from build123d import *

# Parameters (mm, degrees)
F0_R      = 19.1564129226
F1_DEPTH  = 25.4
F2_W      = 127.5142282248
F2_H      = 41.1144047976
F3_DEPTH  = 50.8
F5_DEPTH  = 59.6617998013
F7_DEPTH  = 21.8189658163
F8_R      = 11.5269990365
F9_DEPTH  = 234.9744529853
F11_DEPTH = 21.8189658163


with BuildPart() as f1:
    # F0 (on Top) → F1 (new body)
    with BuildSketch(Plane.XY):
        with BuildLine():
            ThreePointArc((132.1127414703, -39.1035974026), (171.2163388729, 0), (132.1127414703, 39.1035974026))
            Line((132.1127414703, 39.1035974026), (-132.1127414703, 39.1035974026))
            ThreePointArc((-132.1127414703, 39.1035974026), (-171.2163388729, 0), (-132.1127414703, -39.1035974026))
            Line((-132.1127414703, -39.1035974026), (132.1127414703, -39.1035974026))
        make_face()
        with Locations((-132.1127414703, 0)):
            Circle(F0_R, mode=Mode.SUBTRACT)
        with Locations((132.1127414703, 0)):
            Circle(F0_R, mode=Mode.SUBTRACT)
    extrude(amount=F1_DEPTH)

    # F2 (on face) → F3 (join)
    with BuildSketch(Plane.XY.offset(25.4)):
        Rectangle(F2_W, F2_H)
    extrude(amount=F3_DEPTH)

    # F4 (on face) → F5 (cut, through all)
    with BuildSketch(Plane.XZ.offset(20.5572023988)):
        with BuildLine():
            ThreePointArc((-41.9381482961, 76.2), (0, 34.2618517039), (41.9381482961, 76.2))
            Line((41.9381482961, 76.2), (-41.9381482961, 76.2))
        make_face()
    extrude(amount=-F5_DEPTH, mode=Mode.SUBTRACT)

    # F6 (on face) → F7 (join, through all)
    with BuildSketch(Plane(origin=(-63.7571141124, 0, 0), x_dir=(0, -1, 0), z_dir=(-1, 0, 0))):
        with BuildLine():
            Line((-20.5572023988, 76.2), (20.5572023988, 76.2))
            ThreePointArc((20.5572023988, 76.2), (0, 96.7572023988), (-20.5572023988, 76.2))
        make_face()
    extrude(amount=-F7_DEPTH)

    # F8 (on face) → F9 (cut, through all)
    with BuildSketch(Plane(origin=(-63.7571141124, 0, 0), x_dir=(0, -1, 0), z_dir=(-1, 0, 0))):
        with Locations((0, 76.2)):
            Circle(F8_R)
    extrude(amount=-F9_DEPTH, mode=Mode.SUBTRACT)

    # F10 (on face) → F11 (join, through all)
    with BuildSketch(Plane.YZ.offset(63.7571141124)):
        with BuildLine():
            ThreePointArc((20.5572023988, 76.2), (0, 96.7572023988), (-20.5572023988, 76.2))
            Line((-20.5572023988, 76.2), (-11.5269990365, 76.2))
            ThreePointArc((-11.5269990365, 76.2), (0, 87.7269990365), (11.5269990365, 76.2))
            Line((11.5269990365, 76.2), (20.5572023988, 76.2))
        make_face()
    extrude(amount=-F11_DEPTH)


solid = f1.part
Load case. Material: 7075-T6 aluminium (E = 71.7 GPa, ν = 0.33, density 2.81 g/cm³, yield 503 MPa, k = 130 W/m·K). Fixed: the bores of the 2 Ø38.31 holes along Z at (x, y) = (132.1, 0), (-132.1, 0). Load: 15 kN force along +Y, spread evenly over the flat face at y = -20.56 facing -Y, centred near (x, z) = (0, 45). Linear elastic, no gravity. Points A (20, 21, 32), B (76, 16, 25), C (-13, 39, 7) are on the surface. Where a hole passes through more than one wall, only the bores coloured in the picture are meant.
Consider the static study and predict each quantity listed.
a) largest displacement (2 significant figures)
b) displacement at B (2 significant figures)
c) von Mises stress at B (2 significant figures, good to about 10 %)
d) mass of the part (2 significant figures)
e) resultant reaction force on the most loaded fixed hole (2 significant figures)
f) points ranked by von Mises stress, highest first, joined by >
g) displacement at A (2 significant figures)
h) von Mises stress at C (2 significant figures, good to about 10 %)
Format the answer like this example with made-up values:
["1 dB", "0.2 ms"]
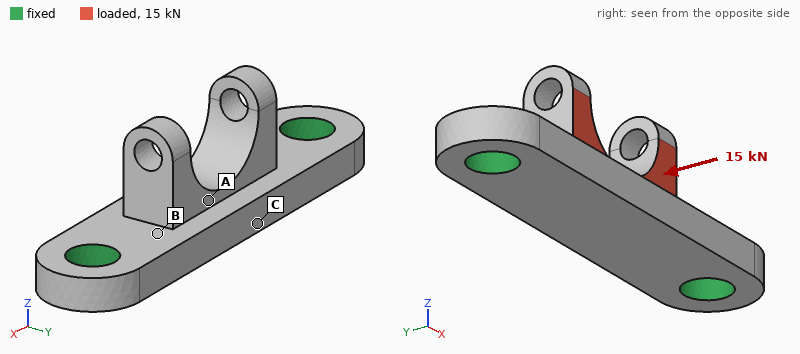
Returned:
["0.16 mm", "0.030 mm", "30 MPa", "2.1 kg", "7.5 kN", "B > C > A", "0.063 mm", "10 MPa"]
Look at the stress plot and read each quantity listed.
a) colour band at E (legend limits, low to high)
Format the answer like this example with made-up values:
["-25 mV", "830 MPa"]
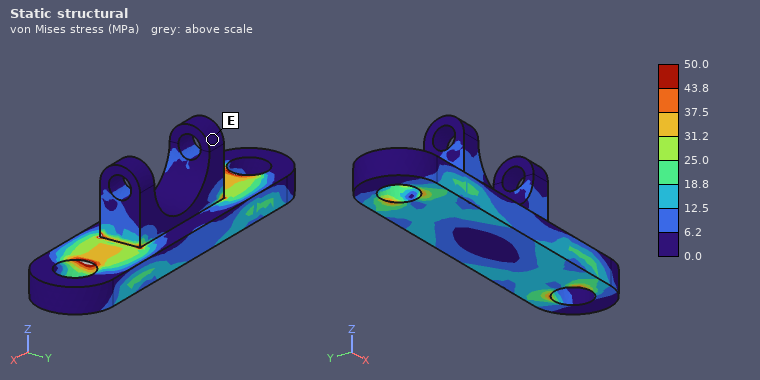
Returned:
["0.0 to 6.2 MPa"]
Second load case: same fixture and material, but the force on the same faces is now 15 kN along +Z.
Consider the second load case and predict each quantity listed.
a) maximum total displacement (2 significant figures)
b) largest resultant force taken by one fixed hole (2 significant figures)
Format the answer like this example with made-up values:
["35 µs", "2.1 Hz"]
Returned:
["0.12 mm", "8.2 kN"]
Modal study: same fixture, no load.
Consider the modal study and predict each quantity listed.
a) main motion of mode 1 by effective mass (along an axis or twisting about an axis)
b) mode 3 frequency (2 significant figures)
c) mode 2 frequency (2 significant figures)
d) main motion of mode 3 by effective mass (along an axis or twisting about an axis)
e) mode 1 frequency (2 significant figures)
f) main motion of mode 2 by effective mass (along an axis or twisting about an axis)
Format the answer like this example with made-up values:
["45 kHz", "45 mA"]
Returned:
["along Z", "3800 Hz", "2300 Hz", "along Y", "2100 Hz", "along Y"]
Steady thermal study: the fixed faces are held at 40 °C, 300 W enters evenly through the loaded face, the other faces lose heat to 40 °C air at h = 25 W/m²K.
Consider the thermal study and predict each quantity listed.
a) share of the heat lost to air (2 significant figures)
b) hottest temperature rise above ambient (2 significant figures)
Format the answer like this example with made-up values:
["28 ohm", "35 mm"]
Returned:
["17 %", "60 K"]
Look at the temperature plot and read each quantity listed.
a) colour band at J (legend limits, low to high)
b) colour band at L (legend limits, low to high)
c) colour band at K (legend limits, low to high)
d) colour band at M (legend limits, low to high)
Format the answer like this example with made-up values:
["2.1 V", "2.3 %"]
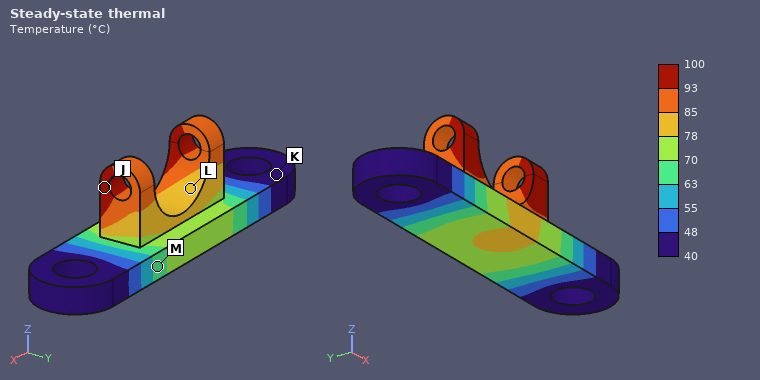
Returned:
["93 to 100 °C", "78 to 85 °C", "40 to 48 °C", "63 to 70 °C"]
